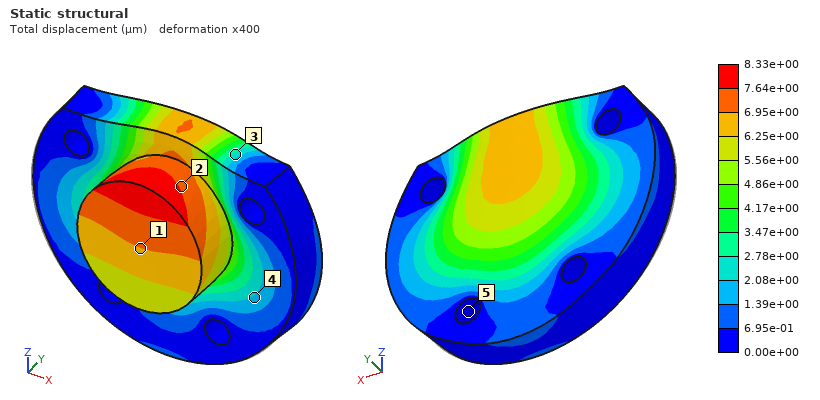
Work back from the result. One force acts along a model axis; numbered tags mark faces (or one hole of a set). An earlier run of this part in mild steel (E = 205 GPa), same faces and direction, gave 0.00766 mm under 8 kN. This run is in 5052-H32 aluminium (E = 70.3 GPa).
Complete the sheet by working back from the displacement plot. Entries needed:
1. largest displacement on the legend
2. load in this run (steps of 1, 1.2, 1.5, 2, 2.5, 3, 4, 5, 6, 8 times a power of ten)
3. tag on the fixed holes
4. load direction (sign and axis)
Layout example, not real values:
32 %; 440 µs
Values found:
8.33e+00 µm; 3 kN; 5; +Y
